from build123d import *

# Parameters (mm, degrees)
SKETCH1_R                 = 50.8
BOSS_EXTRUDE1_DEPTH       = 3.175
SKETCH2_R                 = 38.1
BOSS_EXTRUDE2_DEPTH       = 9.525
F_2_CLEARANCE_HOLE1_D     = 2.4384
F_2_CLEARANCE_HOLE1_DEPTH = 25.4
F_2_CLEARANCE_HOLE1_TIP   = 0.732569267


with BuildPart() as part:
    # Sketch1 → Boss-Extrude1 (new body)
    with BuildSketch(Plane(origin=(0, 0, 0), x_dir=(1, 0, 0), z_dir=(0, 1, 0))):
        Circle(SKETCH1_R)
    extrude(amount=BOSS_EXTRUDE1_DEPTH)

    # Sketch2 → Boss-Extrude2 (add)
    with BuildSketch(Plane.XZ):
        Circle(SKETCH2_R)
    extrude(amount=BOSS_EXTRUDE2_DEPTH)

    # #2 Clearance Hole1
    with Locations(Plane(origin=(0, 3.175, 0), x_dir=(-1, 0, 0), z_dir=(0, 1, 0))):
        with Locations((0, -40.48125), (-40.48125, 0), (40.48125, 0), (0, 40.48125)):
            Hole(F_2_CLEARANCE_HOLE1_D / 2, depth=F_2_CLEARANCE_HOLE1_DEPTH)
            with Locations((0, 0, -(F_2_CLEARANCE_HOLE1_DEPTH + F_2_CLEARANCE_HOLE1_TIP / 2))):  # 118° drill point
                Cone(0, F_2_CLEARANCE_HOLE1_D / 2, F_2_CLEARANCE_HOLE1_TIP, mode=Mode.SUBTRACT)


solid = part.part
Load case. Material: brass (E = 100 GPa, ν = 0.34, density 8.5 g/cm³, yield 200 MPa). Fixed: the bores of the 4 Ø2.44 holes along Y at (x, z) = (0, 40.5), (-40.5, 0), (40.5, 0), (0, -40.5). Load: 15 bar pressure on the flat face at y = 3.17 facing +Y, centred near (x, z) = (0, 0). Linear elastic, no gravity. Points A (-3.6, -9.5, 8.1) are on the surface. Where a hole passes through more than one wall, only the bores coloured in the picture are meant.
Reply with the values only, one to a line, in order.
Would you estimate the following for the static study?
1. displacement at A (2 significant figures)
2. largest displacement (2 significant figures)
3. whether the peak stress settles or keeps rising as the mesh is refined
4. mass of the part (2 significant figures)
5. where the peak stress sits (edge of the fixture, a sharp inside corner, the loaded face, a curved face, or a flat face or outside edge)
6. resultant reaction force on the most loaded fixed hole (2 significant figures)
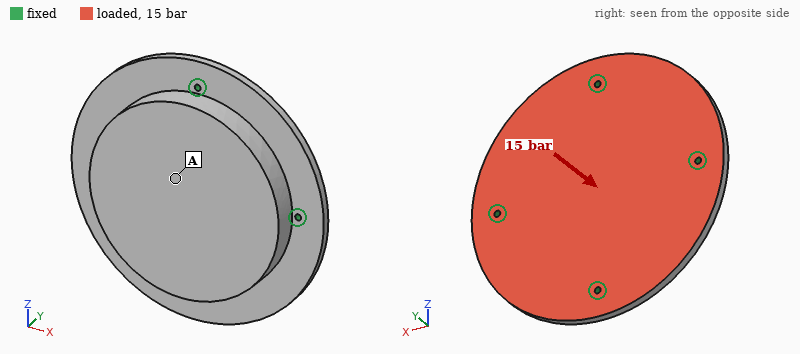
26 µm
58 µm
keeps rising
590 g
edge of the fixture
3.4 kN
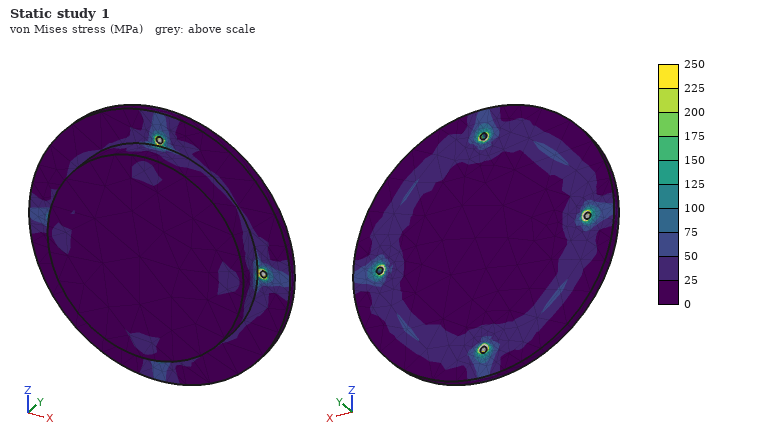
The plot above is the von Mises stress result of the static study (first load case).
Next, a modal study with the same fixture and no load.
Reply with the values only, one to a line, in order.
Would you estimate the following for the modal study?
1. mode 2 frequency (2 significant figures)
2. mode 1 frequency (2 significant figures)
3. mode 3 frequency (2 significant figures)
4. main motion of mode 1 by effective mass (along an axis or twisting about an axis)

5200 Hz
4300 Hz
5200 Hz
along Y
